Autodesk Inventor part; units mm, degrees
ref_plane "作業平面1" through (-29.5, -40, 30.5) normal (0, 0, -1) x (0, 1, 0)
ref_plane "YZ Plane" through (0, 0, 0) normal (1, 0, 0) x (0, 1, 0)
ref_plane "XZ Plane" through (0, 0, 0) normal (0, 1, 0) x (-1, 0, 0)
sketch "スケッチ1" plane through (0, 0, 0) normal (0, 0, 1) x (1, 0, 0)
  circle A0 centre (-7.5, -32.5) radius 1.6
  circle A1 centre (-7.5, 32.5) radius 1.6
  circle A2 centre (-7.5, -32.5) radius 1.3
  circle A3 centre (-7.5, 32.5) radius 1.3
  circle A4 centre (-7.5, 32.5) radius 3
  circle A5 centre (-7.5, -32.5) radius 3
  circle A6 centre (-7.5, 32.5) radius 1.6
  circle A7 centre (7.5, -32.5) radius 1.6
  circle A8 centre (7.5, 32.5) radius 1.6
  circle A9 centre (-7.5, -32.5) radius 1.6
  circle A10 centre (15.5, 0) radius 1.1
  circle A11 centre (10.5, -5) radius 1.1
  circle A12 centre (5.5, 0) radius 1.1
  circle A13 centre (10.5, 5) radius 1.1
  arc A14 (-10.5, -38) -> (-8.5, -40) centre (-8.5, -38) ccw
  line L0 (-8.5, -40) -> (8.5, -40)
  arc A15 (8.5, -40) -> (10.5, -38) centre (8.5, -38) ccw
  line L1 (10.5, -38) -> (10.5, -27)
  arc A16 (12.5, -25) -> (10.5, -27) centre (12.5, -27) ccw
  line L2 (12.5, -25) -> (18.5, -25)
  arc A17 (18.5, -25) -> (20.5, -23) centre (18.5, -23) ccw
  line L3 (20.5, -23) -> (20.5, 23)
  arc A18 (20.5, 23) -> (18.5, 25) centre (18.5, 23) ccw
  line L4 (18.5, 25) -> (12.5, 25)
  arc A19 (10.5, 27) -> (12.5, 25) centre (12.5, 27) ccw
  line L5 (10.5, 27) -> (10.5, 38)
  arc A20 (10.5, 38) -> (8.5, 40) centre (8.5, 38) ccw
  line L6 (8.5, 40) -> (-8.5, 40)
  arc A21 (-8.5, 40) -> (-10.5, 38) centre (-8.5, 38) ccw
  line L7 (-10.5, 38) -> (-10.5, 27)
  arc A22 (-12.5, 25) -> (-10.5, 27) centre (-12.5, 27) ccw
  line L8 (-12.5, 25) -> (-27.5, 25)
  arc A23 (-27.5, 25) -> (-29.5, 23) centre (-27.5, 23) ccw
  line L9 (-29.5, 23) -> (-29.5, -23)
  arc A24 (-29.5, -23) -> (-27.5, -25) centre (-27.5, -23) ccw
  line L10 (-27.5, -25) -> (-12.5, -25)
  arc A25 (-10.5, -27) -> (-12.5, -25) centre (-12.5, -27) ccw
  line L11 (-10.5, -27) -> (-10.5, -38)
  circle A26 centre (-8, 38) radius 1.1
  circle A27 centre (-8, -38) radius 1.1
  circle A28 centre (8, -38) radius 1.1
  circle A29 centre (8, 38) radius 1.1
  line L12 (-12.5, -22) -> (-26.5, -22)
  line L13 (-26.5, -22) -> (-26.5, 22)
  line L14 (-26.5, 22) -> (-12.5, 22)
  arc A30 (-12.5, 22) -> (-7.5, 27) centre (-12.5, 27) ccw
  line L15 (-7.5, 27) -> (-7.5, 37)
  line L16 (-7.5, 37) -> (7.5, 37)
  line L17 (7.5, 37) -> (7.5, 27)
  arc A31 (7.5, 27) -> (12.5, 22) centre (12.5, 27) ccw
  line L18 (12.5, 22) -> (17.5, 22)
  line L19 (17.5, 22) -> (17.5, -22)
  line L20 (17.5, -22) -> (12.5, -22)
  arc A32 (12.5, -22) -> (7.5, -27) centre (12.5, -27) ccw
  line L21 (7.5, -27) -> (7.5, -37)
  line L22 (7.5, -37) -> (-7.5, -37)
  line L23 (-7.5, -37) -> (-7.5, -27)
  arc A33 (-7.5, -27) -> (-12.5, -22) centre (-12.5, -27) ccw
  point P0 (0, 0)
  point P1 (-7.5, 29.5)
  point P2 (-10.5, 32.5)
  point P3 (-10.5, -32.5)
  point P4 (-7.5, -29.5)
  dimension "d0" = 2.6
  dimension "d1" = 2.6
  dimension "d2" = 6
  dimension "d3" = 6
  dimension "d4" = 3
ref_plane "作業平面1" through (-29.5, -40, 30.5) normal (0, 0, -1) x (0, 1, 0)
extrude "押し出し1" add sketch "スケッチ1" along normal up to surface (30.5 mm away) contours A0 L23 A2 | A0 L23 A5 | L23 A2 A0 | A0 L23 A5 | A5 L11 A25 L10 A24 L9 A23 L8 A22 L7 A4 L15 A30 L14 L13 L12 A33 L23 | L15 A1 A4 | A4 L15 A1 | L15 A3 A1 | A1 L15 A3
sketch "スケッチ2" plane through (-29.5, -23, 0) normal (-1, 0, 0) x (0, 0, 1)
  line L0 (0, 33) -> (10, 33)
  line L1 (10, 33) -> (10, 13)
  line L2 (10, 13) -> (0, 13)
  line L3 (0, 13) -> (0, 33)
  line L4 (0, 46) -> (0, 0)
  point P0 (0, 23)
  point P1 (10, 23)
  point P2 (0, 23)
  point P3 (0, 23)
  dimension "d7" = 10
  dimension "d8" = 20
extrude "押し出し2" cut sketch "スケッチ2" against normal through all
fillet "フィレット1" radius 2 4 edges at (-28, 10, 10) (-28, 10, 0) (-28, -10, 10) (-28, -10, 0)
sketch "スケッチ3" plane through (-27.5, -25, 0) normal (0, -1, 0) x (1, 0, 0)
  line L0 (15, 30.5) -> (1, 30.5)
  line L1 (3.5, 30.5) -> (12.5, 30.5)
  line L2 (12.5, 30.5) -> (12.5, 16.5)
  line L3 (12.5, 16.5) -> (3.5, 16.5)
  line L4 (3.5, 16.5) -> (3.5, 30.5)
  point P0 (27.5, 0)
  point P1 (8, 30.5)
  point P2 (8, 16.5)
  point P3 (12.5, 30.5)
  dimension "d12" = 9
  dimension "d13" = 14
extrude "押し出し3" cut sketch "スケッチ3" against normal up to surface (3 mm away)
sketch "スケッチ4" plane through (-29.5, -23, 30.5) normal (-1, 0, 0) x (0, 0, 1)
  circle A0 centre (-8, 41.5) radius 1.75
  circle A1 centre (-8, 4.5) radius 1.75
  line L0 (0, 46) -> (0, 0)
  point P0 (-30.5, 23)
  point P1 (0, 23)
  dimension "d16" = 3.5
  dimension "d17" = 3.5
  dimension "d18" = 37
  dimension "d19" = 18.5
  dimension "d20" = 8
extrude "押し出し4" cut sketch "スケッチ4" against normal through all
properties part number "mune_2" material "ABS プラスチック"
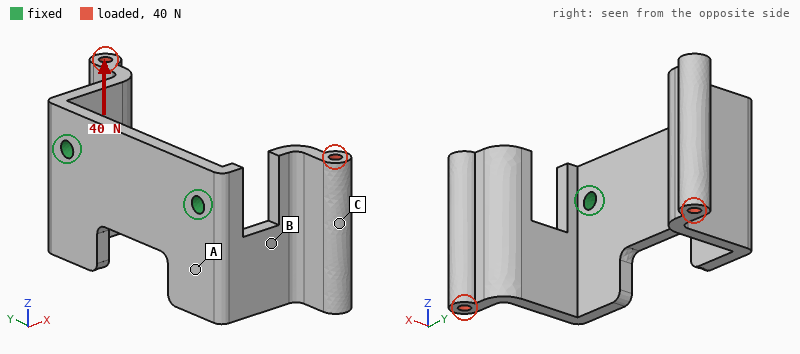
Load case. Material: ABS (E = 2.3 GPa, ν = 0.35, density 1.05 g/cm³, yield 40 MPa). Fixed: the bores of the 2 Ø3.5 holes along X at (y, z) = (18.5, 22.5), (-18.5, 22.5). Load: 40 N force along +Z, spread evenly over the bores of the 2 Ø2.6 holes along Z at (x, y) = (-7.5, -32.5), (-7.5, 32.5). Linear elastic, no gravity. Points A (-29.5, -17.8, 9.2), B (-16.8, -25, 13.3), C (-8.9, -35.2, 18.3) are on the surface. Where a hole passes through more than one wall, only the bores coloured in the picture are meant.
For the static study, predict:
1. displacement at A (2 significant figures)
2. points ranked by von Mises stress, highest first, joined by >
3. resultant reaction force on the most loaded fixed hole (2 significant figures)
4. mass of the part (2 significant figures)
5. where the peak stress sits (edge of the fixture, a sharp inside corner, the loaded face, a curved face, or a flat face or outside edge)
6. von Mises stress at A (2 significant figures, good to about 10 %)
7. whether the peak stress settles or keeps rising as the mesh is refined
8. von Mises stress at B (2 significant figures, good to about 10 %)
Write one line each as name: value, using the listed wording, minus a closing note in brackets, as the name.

displacement at A: 0.21 mm
points ranked by von Mises stress, highest first, joined by >: B > A > C
resultant reaction force on the most loaded fixed hole: 22 N
mass of the part: 9.5 g
where the peak stress sits: edge of the fixture
von Mises stress at A: 3.3 MPa
whether the peak stress settles or keeps rising as the mesh is refined: keeps rising
von Mises stress at B: 7.1 MPa
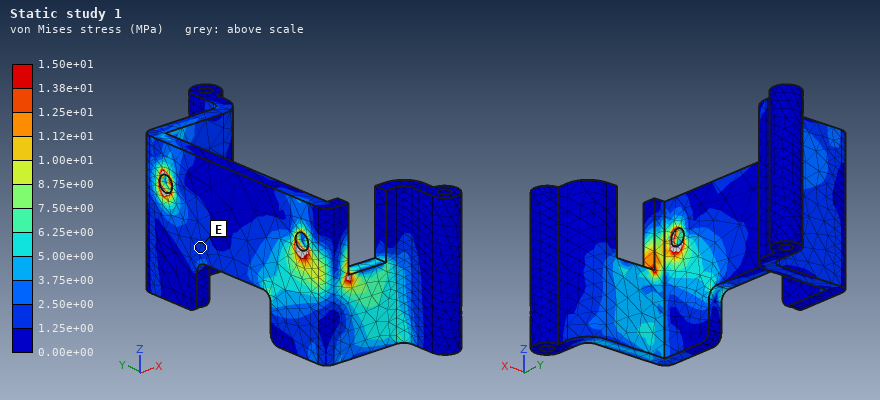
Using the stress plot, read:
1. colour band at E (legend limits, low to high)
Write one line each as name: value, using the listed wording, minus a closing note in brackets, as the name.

colour band at E: 1.25e+00 to 2.50e+00 MPa
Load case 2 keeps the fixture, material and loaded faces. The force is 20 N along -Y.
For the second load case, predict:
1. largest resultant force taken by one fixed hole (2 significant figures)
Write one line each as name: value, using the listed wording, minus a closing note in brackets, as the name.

largest resultant force taken by one fixed hole: 12 N
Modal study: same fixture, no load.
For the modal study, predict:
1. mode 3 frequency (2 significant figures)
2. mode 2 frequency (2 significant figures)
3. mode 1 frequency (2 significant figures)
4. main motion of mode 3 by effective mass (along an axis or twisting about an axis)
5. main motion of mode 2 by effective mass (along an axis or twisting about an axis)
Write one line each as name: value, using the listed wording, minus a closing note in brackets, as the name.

mode 3 frequency: 660 Hz
mode 2 frequency: 610 Hz
mode 1 frequency: 450 Hz
main motion of mode 3 by effective mass: along Z
main motion of mode 2 by effective mass: along Y
